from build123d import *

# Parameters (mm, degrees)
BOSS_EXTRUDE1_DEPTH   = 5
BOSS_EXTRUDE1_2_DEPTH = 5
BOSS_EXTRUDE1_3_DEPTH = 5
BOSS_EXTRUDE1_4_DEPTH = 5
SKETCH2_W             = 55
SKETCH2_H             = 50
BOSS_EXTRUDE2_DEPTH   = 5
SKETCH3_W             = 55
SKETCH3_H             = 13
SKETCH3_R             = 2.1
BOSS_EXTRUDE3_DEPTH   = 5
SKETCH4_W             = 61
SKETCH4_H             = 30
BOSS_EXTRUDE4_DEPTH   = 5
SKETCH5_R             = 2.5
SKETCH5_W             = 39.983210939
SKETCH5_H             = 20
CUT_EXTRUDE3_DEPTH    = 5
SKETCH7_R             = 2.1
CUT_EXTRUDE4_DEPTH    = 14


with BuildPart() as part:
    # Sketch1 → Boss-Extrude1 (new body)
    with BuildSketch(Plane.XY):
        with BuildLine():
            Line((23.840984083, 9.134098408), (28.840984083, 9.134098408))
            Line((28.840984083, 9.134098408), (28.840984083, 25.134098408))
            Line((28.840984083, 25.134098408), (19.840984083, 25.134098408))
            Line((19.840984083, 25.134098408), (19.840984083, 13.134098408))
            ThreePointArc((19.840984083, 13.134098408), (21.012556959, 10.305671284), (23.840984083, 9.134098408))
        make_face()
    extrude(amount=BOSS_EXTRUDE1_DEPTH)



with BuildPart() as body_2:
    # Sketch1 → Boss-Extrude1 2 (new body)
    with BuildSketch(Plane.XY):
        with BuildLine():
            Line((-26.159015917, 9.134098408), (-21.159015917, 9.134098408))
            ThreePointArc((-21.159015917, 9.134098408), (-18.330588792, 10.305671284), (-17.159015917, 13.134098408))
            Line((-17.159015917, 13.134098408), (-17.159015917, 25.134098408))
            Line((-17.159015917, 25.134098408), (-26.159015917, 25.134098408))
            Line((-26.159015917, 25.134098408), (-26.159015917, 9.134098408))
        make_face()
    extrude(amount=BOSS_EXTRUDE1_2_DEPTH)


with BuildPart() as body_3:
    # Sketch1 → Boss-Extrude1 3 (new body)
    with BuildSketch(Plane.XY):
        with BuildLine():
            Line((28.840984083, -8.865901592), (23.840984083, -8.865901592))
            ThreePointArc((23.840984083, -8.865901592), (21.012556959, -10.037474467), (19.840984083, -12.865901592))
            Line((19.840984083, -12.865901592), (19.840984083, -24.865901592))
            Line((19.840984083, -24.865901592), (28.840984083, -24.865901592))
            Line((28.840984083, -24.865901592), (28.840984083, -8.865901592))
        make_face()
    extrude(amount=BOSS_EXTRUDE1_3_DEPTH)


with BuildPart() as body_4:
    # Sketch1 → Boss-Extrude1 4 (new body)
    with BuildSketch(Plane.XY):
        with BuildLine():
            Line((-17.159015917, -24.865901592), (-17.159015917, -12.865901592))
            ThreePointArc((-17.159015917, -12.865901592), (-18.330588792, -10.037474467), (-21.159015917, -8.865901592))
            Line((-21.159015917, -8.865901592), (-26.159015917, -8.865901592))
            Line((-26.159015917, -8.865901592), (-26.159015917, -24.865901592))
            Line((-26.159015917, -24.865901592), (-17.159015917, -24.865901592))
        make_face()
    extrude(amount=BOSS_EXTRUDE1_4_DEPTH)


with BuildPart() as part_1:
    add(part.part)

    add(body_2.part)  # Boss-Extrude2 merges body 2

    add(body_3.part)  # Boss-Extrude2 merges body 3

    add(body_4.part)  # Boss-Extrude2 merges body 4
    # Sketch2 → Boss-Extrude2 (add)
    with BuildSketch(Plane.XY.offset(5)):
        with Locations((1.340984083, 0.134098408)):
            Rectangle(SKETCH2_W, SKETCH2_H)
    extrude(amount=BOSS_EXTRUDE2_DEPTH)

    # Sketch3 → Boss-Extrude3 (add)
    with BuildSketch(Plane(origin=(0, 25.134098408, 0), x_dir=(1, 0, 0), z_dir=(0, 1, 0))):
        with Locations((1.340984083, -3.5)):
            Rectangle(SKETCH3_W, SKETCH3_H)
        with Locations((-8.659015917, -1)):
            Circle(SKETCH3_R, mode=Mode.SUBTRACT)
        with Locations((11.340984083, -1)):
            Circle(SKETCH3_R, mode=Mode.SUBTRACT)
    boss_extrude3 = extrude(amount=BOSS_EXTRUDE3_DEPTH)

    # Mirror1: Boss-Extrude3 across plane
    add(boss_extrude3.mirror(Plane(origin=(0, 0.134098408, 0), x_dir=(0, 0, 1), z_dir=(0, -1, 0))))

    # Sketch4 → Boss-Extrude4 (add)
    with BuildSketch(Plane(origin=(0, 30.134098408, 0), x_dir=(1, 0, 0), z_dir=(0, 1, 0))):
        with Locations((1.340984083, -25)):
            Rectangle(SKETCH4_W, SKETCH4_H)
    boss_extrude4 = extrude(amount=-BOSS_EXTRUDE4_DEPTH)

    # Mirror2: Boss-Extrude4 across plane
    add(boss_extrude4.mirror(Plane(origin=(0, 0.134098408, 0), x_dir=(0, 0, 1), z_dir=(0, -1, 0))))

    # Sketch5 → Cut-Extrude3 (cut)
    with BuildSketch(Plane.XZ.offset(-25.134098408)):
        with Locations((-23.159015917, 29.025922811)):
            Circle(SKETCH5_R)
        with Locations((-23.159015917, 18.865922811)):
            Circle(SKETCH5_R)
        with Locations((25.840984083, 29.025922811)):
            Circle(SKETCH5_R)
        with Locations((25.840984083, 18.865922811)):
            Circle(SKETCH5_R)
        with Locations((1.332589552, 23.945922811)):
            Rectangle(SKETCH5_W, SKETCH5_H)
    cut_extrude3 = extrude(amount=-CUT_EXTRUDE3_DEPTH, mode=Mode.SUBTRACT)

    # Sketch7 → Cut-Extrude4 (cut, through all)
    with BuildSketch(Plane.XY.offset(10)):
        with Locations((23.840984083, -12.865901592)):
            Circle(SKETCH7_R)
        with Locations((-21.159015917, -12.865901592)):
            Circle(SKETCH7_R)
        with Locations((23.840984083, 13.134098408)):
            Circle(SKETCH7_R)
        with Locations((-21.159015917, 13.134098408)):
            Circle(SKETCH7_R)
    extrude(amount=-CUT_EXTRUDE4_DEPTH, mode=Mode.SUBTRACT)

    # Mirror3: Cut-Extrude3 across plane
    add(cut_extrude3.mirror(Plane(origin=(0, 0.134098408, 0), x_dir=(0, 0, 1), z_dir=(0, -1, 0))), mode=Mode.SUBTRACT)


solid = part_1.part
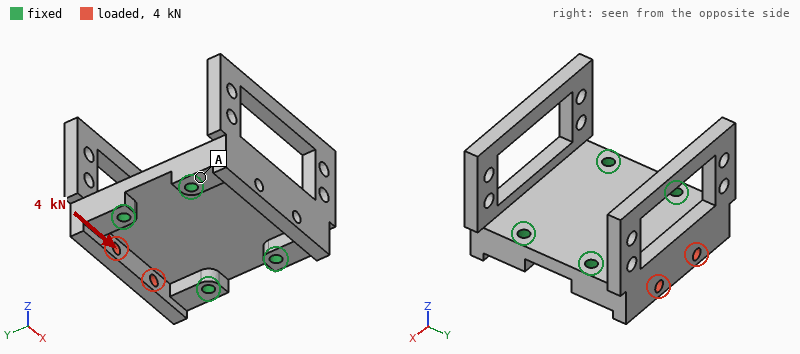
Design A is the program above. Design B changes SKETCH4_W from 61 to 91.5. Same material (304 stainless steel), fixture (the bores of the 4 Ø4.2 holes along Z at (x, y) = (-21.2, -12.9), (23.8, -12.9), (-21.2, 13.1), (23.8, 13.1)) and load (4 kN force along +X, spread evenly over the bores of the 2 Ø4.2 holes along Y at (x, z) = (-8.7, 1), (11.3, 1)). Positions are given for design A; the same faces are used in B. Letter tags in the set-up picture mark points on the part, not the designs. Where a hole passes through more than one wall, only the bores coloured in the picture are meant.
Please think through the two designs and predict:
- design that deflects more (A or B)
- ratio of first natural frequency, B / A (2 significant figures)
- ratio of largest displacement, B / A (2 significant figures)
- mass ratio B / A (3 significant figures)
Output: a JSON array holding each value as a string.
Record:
["B", "0.84", "1.4", "1.28"]
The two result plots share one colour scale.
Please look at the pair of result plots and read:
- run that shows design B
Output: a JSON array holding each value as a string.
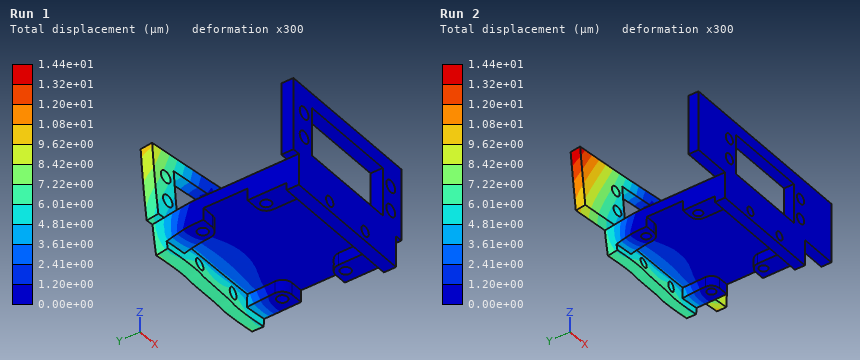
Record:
["Run 2"]
